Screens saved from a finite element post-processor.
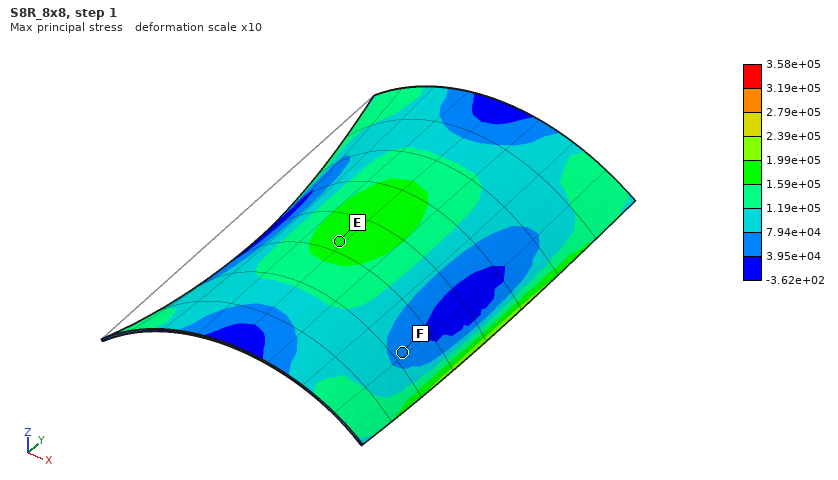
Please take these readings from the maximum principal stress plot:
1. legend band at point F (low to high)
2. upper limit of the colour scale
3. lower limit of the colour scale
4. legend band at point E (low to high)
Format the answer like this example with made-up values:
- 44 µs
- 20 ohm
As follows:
- 3.95e+04 to 7.94e+04
- 3.58e+05
- -3.62e+02
- 1.59e+05 to 1.99e+05
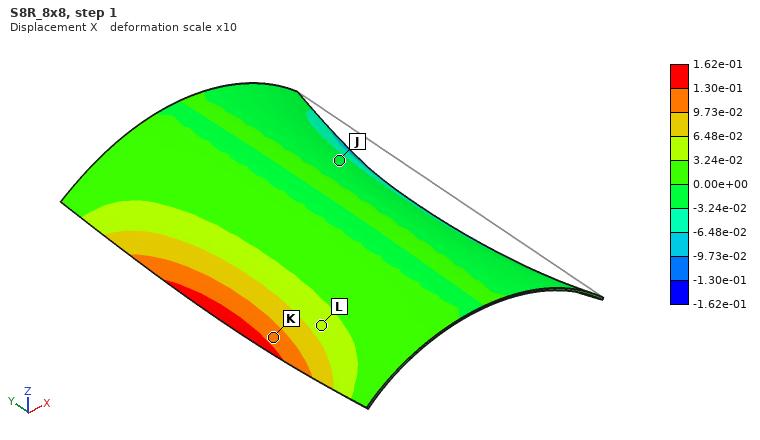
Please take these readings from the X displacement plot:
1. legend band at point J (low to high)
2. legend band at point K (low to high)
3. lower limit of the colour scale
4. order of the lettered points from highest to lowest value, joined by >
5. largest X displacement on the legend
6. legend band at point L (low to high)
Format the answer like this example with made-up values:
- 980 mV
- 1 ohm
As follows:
- -3.24e-02 to 0.00e+00
- 9.73e-02 to 1.30e-01
- -1.62e-01
- K > L > J
- 1.62e-01
- 3.24e-02 to 6.48e-02
